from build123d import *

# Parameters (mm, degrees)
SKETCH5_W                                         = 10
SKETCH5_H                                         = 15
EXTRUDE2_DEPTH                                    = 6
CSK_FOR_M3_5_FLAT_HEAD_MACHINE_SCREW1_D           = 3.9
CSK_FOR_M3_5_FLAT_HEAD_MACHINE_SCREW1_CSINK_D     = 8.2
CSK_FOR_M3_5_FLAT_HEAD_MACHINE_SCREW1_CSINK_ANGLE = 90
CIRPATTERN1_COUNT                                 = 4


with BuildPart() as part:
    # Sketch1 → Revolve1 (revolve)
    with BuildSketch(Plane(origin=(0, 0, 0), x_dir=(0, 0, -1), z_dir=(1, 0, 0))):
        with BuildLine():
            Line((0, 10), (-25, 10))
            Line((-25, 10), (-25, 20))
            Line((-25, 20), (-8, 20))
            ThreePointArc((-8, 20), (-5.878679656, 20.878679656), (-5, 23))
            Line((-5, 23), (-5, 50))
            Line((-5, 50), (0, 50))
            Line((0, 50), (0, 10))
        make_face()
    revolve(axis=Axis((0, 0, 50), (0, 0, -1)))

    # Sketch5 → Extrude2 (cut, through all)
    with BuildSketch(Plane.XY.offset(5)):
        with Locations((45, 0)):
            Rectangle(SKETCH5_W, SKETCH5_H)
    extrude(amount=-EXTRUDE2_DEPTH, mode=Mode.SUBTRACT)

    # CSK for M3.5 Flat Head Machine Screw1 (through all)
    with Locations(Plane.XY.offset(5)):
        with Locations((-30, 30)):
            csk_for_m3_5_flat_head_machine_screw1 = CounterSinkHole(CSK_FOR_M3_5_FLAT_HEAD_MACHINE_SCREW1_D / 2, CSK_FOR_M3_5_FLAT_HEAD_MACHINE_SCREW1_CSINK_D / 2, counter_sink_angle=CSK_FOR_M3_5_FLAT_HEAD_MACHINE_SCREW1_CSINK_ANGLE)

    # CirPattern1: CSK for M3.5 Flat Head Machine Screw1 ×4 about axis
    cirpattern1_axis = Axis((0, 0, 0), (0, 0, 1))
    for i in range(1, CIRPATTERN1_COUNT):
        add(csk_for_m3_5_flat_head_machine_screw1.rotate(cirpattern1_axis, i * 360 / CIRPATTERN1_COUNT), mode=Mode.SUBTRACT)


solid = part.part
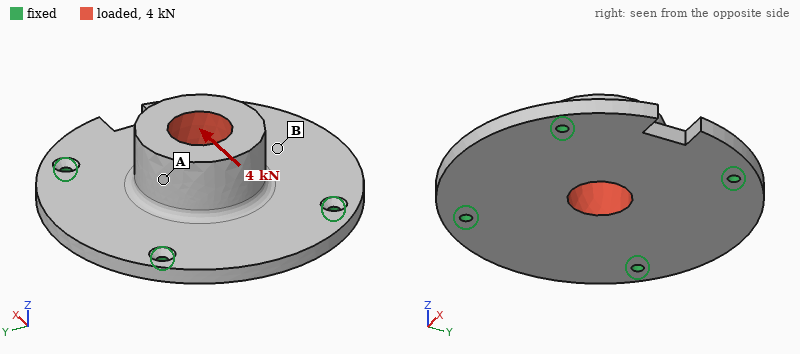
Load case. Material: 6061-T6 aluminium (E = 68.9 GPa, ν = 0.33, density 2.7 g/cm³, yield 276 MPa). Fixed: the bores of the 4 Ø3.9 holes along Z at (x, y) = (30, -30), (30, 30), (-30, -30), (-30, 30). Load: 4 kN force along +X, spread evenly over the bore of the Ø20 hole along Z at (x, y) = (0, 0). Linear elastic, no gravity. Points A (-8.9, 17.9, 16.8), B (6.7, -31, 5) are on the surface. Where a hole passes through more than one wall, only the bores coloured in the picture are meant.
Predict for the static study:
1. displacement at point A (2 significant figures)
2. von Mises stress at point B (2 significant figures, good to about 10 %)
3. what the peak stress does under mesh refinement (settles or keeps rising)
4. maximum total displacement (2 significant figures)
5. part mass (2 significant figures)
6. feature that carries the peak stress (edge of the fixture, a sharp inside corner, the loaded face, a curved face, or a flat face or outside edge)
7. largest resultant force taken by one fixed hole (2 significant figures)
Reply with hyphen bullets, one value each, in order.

- 24 µm
- 15 MPa
- keeps rising
- 41 µm
- 150 g
- edge of the fixture
- 1.2 kN
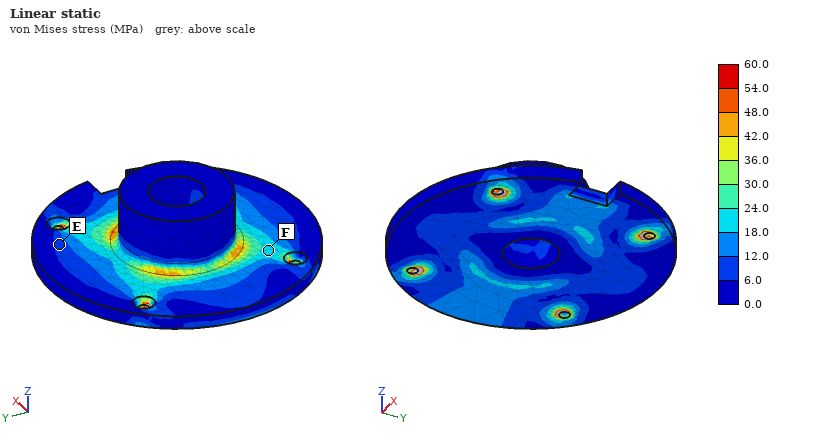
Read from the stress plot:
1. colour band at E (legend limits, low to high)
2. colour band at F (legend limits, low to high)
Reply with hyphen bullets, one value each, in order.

- 6.0 to 12.0 MPa
- 18.0 to 24.0 MPa
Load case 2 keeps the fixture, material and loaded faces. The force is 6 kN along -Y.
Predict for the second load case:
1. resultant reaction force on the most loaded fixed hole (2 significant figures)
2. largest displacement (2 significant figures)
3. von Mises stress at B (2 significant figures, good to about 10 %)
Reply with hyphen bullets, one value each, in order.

- 1.7 kN
- 60 µm
- 21 MPa
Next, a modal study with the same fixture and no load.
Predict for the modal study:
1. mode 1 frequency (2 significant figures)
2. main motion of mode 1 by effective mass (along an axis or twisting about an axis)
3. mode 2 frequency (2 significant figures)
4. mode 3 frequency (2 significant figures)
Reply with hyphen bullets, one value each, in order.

- 3700 Hz
- along Z
- 4700 Hz
- 4800 Hz
